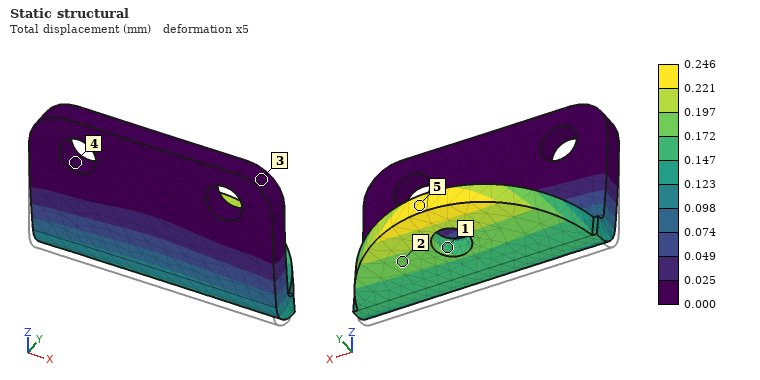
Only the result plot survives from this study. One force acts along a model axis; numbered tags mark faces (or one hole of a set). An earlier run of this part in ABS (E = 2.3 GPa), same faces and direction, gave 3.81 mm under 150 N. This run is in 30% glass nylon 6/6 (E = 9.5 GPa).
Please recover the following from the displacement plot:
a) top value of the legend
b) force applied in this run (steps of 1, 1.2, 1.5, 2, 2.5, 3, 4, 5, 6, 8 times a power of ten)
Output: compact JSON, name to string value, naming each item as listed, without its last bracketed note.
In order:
{"top value of the legend": "0.246 mm", "force applied in this run": "40 N"}
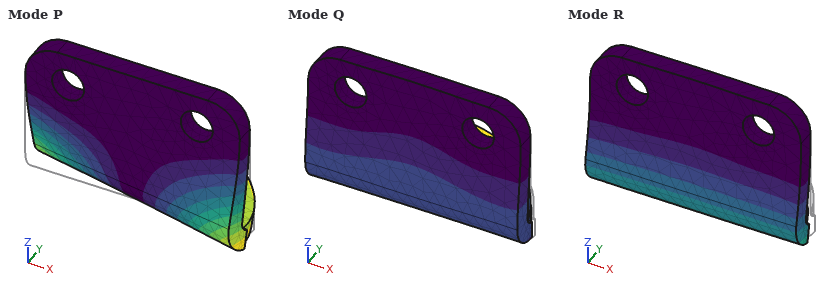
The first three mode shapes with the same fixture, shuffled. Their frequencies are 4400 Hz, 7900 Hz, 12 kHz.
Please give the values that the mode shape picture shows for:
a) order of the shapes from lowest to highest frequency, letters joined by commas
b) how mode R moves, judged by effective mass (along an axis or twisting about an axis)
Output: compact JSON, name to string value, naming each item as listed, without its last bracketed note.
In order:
{"order of the shapes from lowest to highest frequency, letters joined by commas": "R, P, Q", "how mode R moves, judged by effective mass": "along Y"}
